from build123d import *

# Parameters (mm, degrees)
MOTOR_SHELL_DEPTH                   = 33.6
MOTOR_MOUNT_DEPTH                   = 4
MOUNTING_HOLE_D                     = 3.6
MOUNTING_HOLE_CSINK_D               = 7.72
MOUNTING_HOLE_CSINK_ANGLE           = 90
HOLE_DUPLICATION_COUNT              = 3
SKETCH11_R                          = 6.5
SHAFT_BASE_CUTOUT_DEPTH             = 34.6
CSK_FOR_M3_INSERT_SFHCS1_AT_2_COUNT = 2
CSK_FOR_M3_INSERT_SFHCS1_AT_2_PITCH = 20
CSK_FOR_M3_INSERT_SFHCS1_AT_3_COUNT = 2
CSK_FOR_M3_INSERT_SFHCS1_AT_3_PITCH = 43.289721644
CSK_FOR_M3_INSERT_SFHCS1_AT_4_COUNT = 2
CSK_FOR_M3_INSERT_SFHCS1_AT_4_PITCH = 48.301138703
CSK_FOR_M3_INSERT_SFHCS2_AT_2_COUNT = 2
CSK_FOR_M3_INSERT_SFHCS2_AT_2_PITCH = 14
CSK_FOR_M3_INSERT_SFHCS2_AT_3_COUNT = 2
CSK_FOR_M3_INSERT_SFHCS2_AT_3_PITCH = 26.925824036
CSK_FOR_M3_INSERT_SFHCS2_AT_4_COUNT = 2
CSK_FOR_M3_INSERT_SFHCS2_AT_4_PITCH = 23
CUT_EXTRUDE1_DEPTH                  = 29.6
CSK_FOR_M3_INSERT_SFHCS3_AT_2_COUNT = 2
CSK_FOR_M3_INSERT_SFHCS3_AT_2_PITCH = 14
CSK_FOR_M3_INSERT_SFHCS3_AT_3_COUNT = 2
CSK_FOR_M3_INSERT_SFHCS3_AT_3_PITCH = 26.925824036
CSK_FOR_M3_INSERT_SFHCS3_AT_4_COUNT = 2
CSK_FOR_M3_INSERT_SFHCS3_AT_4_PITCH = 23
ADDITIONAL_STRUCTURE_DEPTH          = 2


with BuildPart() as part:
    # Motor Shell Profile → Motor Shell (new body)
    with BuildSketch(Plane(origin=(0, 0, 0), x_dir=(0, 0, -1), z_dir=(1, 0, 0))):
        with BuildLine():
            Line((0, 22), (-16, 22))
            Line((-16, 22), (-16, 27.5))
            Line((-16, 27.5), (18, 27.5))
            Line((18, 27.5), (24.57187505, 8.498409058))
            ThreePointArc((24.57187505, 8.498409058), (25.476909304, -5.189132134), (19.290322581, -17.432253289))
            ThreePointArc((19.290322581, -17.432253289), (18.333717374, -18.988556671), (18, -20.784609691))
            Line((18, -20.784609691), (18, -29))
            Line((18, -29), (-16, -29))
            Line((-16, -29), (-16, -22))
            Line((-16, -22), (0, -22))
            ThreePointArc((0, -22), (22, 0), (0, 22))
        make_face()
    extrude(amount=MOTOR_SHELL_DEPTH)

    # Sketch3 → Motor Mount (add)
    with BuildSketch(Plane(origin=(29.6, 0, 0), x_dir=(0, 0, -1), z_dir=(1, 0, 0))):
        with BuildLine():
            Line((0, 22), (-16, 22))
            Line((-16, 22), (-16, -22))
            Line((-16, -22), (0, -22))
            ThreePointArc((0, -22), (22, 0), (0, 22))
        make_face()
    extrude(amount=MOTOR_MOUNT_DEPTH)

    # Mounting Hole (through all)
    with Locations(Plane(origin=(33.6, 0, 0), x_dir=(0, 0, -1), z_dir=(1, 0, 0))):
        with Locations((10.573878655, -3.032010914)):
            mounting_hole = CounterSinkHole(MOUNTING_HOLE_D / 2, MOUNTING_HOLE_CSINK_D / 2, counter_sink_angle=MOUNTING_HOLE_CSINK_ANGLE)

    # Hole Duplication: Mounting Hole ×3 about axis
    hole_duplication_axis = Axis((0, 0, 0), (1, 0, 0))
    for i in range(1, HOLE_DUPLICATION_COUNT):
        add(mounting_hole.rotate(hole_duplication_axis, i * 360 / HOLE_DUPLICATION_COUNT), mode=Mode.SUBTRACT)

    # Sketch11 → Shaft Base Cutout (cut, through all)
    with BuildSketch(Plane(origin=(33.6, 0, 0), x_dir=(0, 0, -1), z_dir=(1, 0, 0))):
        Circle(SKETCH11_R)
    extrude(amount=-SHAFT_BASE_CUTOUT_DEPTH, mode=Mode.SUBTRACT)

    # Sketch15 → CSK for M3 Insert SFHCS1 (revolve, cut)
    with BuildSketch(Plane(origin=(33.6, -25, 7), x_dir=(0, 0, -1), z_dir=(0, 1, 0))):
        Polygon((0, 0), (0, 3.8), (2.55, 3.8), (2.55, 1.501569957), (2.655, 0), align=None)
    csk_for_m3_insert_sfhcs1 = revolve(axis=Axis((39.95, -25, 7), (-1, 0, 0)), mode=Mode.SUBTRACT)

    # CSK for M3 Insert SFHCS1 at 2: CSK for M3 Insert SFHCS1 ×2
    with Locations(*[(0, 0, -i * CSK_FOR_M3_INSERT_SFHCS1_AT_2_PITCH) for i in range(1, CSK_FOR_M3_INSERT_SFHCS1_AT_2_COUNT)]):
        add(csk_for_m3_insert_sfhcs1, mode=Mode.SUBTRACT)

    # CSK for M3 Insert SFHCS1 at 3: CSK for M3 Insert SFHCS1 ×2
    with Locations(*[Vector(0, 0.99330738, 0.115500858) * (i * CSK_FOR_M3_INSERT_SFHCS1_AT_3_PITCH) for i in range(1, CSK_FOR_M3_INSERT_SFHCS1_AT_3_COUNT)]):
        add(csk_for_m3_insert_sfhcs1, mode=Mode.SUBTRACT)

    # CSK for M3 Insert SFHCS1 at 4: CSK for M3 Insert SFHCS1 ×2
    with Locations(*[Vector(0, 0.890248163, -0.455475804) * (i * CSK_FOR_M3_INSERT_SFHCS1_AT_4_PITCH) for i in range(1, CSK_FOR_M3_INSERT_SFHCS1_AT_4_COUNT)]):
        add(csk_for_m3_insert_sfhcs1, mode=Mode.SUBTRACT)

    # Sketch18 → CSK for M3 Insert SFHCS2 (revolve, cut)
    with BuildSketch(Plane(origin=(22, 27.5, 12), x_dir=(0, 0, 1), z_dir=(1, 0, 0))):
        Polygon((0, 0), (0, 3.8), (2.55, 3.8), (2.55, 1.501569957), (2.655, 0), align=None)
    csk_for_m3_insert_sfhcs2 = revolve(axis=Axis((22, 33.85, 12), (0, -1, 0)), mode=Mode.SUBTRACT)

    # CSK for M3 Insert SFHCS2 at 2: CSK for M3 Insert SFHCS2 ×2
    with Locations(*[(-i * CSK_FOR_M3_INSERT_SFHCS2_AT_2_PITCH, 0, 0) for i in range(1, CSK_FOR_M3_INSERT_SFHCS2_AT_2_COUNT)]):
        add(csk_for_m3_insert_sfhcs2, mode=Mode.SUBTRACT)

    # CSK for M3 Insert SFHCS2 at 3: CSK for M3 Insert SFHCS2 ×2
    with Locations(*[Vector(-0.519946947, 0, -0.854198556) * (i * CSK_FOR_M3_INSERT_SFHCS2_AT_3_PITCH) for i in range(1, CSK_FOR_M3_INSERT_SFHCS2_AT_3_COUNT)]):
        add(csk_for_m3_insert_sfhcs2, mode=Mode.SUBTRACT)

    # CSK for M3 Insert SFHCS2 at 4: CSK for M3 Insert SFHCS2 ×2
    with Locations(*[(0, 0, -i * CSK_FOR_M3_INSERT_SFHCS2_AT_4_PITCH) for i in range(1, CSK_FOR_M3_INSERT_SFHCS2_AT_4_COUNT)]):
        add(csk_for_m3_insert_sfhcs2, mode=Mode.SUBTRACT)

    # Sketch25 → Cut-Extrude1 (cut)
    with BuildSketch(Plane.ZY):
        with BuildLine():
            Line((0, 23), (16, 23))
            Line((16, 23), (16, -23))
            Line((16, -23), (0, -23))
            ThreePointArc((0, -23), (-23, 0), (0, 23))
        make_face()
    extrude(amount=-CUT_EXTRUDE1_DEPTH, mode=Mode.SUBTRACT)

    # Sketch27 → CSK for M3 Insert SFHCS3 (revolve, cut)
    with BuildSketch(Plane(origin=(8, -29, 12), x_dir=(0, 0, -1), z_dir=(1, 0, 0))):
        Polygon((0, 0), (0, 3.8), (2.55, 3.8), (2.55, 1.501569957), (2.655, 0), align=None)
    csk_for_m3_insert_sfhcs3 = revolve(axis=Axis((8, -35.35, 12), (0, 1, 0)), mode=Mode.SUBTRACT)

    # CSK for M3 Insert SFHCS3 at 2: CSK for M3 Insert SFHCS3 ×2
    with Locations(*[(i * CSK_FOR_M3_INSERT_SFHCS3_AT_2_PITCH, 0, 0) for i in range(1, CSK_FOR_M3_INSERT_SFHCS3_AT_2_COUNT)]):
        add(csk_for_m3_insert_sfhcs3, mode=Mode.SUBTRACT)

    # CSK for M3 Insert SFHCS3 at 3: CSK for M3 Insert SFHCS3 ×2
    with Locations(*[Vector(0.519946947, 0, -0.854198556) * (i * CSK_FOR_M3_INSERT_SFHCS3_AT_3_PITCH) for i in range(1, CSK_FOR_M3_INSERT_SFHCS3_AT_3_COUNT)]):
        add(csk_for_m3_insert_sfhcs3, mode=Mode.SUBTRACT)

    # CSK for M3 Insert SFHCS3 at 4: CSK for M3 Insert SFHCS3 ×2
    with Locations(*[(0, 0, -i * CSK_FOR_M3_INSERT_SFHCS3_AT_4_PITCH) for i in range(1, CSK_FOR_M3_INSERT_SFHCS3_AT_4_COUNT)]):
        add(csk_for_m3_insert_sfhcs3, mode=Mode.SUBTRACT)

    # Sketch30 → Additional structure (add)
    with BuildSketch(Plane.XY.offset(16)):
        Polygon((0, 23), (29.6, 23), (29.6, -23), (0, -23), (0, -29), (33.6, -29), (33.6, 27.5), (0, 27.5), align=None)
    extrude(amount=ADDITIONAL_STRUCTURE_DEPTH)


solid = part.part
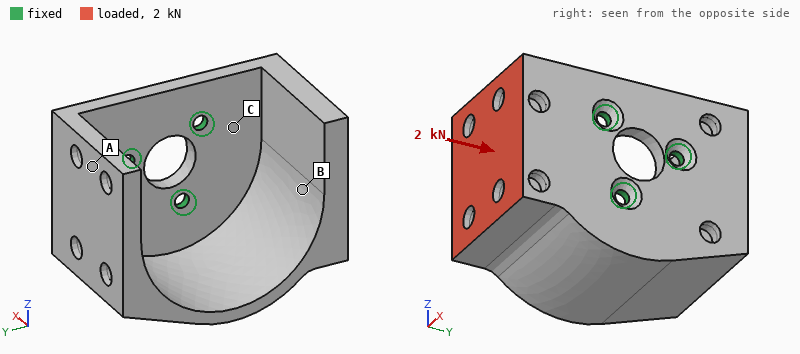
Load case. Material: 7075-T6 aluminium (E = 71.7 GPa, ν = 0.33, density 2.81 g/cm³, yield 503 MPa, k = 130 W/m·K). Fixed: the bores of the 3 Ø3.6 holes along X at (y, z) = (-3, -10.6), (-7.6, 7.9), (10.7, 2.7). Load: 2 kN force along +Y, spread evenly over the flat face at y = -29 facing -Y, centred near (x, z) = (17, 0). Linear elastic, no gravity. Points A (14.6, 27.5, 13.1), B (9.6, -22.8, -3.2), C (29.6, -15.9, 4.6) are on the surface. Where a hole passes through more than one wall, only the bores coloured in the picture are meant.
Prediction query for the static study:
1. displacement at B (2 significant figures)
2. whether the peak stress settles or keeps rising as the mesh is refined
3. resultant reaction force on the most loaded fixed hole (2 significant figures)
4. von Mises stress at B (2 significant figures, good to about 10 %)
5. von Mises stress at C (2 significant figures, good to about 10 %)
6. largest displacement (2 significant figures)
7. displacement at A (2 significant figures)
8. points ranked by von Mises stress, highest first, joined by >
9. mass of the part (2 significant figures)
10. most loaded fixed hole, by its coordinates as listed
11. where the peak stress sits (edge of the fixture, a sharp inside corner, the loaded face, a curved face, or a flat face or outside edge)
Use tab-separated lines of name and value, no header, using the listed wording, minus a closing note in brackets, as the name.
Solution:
displacement at B	0.41 mm
whether the peak stress settles or keeps rising as the mesh is refined	keeps rising
resultant reaction force on the most loaded fixed hole	1.0 kN
von Mises stress at B	49 MPa
von Mises stress at C	110 MPa
largest displacement	0.66 mm
displacement at A	0.20 mm
points ranked by von Mises stress, highest first, joined by >	C > B > A
mass of the part	71 g
most loaded fixed hole, by its coordinates as listed	(-7.6, 7.9)
where the peak stress sits	edge of the fixture
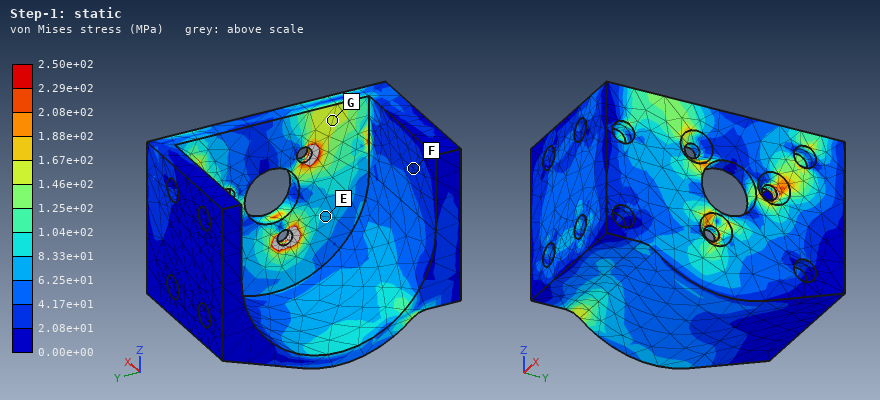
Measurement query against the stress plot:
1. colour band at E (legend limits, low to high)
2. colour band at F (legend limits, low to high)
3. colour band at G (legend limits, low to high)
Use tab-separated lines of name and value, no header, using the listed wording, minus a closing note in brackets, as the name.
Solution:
colour band at E	6.25e+01 to 8.33e+01 MPa
colour band at F	2.08e+01 to 4.17e+01 MPa
colour band at G	1.46e+02 to 1.67e+02 MPa
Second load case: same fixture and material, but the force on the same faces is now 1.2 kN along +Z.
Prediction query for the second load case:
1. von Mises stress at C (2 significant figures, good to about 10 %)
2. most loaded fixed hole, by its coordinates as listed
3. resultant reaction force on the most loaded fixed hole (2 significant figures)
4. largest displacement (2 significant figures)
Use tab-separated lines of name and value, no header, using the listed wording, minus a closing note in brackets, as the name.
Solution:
von Mises stress at C	71 MPa
most loaded fixed hole, by its coordinates as listed	(-3, -10.6)
resultant reaction force on the most loaded fixed hole	1.5 kN
largest displacement	0.18 mm
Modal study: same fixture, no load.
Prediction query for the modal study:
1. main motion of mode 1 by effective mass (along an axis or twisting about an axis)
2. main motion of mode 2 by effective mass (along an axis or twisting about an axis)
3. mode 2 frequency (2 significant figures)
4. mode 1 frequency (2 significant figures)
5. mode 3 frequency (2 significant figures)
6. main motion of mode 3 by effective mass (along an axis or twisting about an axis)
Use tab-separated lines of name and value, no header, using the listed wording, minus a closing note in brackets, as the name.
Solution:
main motion of mode 1 by effective mass	along Y
main motion of mode 2 by effective mass	along Z
mode 2 frequency	2400 Hz
mode 1 frequency	1400 Hz
mode 3 frequency	3400 Hz
main motion of mode 3 by effective mass	along X
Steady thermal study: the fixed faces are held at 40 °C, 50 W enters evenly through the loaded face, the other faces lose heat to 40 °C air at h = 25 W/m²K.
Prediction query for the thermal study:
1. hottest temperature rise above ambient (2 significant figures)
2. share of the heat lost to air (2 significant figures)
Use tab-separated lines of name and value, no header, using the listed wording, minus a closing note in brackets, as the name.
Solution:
hottest temperature rise above ambient	58 K
share of the heat lost to air	12 %
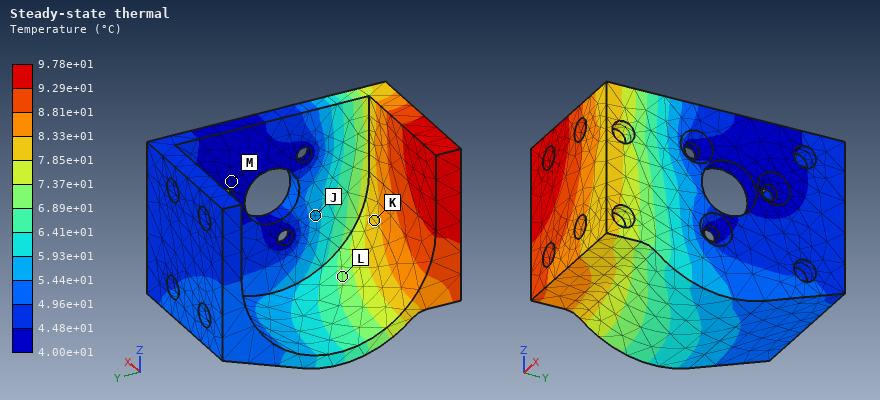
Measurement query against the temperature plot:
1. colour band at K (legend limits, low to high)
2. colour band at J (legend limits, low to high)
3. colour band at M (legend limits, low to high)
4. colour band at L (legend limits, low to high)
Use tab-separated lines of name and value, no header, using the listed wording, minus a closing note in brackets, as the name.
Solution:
colour band at K	7.85e+01 to 8.33e+01 °C
colour band at J	5.44e+01 to 5.93e+01 °C
colour band at M	4.00e+01 to 4.48e+01 °C
colour band at L	6.89e+01 to 7.37e+01 °C
